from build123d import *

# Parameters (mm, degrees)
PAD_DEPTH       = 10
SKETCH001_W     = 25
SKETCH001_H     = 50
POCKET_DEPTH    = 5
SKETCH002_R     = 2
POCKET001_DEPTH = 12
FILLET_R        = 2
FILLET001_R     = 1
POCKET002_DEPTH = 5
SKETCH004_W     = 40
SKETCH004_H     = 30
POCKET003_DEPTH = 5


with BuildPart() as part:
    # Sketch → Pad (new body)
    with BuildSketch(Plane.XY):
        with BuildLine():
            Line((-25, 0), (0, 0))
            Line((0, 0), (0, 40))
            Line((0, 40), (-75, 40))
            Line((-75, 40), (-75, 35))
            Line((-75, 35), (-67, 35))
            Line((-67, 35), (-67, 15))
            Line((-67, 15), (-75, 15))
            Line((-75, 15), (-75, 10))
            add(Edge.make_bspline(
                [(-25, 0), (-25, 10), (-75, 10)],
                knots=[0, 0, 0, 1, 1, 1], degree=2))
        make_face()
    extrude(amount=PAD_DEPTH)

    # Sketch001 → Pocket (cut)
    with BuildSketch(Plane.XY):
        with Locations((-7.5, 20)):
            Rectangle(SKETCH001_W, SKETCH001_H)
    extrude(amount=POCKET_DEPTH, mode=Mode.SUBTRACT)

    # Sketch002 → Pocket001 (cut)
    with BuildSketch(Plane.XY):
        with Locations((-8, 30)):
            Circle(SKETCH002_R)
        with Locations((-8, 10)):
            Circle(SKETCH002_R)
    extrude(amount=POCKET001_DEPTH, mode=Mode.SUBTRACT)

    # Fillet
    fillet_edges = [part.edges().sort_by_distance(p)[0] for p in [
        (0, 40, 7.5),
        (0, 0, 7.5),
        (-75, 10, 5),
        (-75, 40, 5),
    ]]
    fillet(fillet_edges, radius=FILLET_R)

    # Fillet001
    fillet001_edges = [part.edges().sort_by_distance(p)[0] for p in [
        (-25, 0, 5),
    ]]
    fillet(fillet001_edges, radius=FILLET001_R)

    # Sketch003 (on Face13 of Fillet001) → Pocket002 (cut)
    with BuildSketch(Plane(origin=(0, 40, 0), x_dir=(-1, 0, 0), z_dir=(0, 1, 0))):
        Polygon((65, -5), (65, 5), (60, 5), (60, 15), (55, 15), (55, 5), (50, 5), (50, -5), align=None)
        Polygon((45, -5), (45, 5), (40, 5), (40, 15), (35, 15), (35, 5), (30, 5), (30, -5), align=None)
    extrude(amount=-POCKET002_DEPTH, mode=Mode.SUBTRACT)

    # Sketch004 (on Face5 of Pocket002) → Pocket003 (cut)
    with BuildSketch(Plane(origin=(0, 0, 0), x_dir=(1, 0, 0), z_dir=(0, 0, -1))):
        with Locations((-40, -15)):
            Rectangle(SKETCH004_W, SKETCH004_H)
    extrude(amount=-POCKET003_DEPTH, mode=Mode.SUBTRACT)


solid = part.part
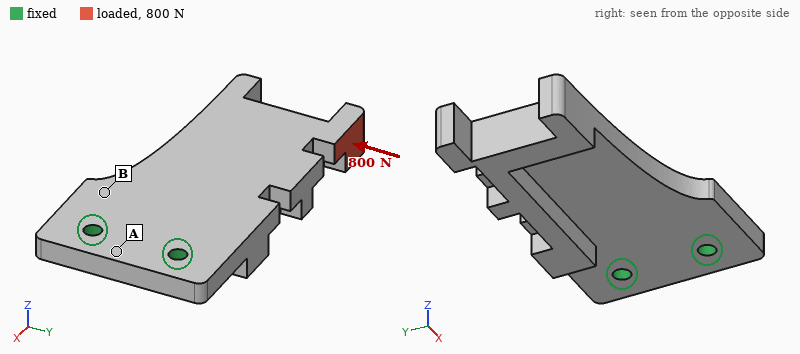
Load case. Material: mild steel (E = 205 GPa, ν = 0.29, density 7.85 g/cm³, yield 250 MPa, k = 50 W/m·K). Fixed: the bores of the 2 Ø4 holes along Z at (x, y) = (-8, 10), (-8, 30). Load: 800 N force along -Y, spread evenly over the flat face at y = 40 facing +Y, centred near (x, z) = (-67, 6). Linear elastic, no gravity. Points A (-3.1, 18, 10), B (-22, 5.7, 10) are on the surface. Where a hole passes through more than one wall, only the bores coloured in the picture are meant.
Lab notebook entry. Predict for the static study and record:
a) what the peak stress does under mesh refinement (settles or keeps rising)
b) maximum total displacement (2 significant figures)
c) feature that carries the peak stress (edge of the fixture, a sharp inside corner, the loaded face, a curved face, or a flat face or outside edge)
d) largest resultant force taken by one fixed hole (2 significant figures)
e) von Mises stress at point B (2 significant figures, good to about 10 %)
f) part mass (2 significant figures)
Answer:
keeps rising
46 µm
edge of the fixture
2.2 kN
24 MPa
110 g
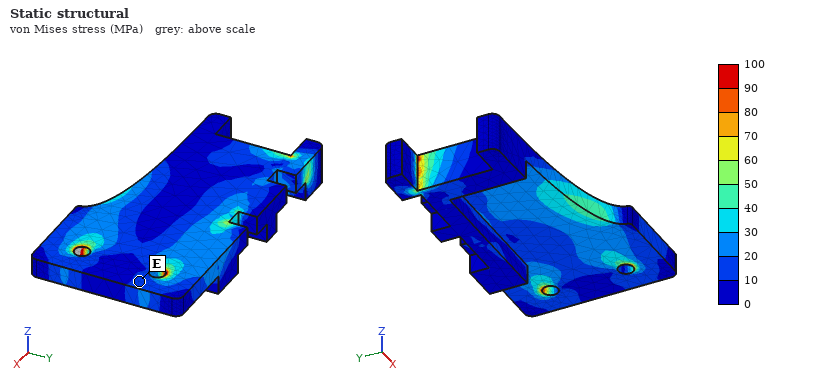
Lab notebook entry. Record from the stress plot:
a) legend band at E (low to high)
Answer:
10 to 20 MPa
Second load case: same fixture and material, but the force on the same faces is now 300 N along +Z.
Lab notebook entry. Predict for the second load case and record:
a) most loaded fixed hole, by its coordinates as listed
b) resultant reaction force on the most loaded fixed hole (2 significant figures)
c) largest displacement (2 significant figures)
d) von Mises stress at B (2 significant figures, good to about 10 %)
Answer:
(-8, 30)
360 N
0.29 mm
64 MPa
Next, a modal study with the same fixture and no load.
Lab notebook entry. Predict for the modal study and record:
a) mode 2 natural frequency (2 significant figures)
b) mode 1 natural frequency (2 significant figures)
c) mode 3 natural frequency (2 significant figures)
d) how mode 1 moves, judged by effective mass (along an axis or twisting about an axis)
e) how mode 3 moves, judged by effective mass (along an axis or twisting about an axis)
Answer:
4000 Hz
1000 Hz
5100 Hz
along Z
along Y
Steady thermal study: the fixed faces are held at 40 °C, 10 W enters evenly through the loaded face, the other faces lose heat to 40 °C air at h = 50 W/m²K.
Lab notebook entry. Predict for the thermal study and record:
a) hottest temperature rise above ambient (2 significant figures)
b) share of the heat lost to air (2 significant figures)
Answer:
69 K
58 %
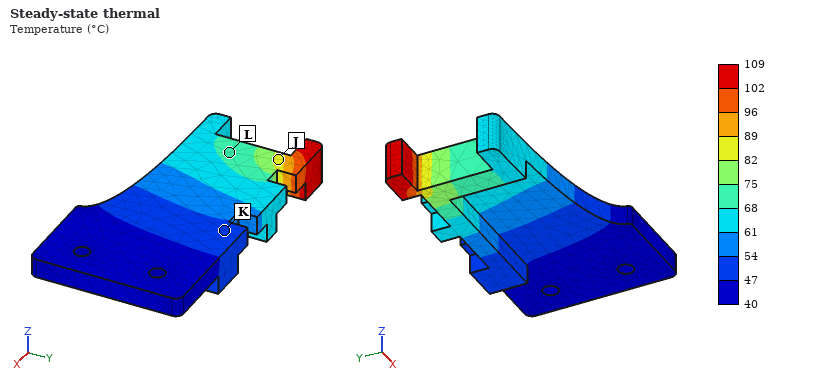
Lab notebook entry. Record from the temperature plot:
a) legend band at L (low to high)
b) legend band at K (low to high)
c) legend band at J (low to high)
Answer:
68 to 75 °C
47 to 54 °C
82 to 89 °C
